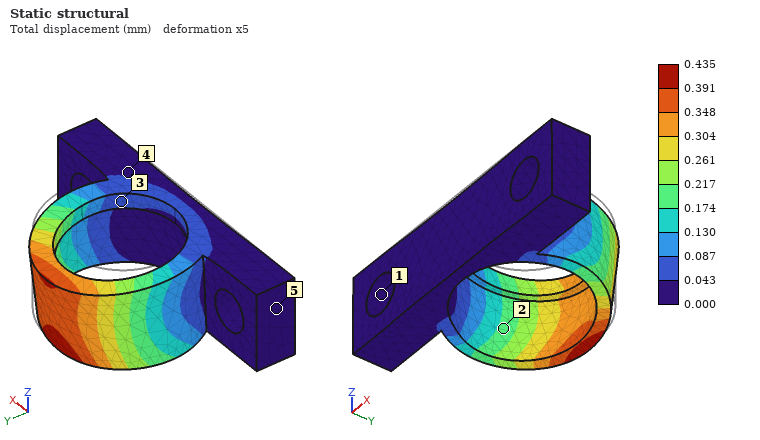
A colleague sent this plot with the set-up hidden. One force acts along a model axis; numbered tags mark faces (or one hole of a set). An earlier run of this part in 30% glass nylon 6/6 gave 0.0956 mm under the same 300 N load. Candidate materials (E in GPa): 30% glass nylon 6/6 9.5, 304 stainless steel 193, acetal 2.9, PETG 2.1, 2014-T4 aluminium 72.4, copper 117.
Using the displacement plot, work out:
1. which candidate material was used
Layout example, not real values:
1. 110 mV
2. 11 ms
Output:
1. PETG
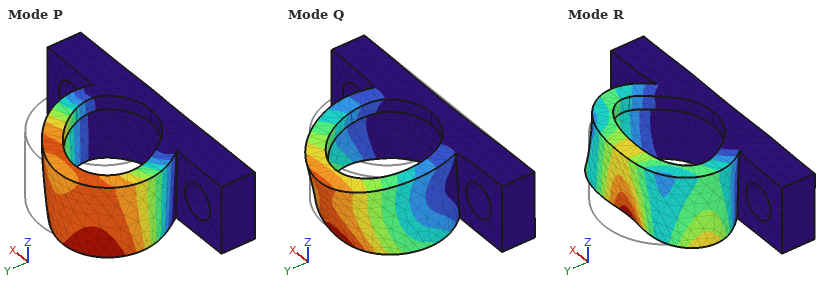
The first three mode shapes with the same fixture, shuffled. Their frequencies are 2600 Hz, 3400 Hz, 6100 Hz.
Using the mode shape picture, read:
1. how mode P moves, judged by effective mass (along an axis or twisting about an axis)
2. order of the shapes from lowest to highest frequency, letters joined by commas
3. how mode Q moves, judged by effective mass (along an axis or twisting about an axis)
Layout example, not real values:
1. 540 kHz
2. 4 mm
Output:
1. along X
2. P, Q, R
3. along Z
